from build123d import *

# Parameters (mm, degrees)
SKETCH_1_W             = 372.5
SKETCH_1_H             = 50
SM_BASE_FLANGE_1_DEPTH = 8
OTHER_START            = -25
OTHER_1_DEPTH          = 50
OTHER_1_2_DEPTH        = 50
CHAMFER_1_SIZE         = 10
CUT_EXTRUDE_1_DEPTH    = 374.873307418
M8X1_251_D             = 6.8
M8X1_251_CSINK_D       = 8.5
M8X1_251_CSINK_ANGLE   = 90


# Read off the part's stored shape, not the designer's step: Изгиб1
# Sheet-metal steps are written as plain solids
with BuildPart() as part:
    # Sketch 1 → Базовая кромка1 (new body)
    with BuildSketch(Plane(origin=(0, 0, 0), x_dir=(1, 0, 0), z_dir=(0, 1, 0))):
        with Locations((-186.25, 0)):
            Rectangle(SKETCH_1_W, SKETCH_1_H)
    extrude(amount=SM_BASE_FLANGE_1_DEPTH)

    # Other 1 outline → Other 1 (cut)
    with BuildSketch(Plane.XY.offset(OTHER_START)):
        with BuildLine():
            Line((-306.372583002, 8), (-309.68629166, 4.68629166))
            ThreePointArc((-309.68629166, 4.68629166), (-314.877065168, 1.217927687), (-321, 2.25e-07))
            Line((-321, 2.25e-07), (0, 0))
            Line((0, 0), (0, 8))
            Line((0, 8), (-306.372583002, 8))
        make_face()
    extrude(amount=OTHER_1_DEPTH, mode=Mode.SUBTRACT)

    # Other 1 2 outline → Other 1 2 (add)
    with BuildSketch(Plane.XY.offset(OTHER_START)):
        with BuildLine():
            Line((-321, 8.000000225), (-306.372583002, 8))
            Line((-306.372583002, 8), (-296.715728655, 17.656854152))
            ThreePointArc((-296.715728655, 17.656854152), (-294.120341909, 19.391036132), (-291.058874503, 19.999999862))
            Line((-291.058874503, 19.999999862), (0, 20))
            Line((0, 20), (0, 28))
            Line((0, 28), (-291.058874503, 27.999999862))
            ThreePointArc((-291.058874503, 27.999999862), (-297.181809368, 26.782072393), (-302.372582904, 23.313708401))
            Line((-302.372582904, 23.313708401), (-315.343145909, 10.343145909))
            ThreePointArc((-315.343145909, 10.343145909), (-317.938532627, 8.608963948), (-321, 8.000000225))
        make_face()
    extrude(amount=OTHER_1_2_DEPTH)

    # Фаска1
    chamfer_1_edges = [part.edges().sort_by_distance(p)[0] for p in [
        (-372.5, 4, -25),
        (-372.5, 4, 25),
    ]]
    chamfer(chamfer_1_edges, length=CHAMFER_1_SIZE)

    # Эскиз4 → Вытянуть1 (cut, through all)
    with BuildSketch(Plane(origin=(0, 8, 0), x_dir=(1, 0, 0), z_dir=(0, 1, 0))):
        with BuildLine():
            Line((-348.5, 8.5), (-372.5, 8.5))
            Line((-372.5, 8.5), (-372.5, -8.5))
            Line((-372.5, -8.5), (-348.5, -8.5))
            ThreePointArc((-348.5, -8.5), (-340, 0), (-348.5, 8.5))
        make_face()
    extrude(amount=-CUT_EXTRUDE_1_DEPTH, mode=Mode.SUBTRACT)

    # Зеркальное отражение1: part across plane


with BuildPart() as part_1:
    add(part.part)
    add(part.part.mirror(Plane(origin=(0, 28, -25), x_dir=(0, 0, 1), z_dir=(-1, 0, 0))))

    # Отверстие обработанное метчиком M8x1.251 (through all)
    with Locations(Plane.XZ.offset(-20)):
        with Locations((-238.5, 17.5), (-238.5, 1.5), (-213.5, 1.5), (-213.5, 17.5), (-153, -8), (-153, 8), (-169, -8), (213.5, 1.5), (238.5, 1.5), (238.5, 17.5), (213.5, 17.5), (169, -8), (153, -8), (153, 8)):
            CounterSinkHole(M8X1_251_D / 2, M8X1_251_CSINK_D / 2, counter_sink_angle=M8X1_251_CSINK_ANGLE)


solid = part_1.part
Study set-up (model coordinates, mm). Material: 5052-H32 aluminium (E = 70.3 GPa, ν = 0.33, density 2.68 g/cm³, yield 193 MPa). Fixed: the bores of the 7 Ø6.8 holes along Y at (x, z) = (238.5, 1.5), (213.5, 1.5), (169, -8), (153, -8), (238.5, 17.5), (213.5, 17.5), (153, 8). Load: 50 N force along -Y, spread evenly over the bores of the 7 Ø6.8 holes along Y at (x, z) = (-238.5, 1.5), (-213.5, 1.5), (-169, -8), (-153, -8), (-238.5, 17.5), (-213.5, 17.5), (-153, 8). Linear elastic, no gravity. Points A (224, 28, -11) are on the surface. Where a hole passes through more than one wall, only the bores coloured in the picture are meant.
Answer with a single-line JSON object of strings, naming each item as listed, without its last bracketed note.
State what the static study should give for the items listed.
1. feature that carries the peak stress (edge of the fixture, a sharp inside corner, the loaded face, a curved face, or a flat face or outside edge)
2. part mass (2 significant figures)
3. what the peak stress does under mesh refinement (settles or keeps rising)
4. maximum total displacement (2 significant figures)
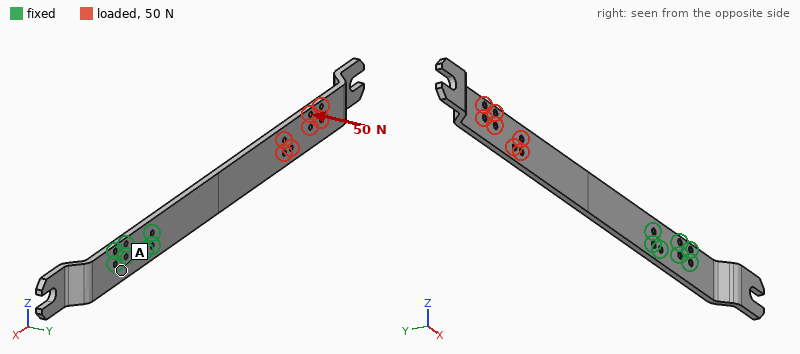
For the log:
{"feature that carries the peak stress": "edge of the fixture", "part mass": "780 g", "what the peak stress does under mesh refinement": "keeps rising", "maximum total displacement": "8.3 mm"}
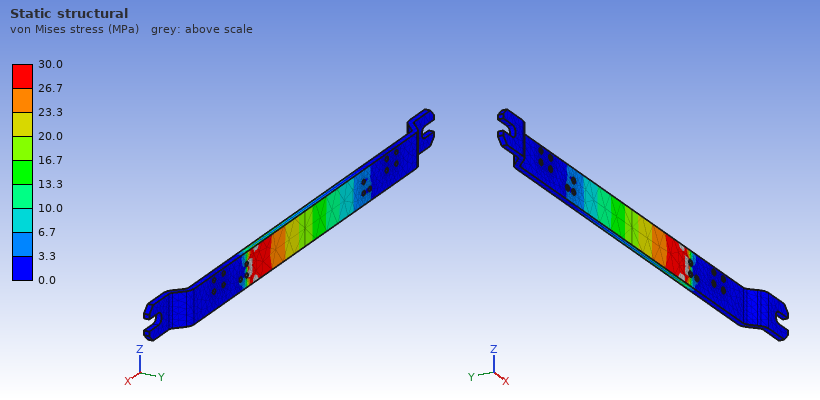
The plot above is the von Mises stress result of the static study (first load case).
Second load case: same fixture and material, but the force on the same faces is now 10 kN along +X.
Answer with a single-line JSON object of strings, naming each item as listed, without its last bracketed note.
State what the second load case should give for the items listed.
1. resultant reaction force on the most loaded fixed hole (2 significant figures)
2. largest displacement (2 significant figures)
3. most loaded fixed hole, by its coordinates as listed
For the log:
{"resultant reaction force on the most loaded fixed hole": "5.7 kN", "largest displacement": "3.6 mm", "most loaded fixed hole, by its coordinates as listed": "(153, 8)"}
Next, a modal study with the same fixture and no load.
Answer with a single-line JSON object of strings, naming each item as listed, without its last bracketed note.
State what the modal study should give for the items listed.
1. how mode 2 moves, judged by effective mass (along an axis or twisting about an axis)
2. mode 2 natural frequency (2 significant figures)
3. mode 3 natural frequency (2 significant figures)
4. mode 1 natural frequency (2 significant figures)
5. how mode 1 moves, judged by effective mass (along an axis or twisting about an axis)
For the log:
{"how mode 2 moves, judged by effective mass": "along Z", "mode 2 natural frequency": "150 Hz", "mode 3 natural frequency": "150 Hz", "mode 1 natural frequency": "25 Hz", "how mode 1 moves, judged by effective mass": "along Y"}
